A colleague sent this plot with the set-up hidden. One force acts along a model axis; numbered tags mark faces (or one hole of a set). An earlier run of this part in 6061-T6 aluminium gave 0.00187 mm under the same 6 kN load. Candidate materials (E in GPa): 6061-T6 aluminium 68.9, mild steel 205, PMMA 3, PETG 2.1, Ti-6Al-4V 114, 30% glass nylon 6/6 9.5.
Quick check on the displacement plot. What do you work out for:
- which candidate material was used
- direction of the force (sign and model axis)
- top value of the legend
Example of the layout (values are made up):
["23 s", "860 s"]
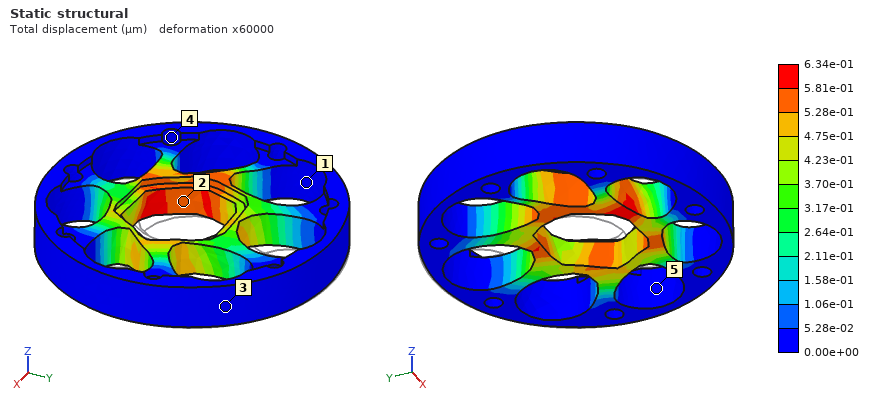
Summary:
["mild steel", "-Y", "6.34e-01 µm"]
